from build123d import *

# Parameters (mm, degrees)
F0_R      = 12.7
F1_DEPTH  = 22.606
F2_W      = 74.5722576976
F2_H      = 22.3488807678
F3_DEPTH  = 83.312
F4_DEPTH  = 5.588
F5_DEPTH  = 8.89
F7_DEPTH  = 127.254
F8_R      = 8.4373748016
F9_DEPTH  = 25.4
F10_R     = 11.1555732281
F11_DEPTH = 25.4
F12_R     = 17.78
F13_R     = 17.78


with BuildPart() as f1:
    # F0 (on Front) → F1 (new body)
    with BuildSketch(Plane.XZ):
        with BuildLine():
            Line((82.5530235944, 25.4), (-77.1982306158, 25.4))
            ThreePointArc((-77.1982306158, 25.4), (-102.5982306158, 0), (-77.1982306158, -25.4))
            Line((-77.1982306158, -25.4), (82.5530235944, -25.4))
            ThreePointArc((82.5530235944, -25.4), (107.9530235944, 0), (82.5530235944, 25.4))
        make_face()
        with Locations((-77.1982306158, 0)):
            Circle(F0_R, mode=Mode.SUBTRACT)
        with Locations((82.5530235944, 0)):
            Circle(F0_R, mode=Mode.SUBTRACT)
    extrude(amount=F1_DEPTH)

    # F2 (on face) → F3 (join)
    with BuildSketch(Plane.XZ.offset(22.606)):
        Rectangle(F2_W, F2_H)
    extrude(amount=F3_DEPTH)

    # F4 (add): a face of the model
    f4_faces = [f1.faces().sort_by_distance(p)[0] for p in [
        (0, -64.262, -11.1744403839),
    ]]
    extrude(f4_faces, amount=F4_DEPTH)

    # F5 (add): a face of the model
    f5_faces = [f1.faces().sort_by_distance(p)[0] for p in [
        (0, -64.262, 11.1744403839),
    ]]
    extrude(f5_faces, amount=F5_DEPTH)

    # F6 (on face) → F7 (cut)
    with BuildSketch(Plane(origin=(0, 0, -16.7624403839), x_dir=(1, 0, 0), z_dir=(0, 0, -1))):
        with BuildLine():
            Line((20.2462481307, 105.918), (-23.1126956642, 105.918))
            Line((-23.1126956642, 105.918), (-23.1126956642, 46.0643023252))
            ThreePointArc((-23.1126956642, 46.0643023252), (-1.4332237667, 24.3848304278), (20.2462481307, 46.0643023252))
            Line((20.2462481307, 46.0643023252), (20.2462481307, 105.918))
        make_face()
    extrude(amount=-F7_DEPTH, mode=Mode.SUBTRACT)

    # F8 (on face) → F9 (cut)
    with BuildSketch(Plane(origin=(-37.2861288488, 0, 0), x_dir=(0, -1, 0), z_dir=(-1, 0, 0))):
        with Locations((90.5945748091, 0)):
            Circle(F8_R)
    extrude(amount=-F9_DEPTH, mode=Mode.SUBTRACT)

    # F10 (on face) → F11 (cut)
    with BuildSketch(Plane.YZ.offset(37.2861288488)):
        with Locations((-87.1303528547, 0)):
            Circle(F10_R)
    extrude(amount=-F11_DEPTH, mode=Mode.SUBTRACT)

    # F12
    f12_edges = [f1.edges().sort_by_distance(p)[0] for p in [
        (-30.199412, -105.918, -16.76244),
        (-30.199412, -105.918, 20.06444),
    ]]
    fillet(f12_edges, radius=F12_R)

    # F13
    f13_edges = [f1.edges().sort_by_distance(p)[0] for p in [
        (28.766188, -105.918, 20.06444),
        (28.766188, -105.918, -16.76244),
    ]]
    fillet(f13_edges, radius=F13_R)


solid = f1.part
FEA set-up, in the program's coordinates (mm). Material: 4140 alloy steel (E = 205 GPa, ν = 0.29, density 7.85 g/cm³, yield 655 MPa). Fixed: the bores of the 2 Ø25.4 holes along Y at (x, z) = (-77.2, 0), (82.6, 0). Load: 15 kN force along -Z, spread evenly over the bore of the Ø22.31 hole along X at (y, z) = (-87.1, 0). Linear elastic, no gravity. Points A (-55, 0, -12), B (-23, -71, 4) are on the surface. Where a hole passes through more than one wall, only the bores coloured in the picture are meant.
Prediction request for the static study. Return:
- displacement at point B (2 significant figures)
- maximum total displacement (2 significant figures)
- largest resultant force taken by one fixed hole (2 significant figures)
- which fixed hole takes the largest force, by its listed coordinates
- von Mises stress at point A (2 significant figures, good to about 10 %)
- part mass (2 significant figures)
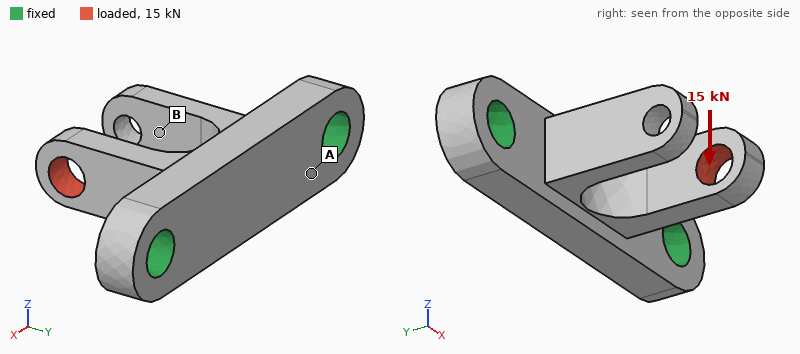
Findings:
0.083 mm
0.41 mm
11 kN
(82.6, 0)
74 MPa
2.3 kg
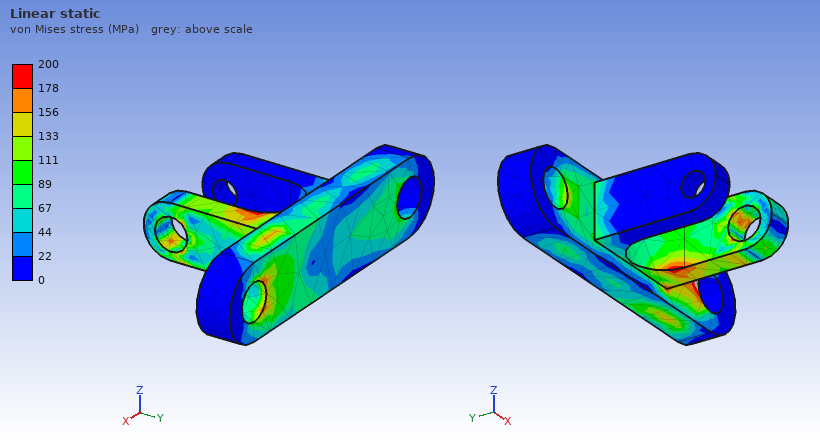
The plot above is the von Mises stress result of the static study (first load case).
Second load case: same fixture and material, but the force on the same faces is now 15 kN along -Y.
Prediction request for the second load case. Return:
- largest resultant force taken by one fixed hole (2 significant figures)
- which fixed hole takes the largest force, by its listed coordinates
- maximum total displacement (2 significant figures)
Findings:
11 kN
(82.6, 0)
34 µm
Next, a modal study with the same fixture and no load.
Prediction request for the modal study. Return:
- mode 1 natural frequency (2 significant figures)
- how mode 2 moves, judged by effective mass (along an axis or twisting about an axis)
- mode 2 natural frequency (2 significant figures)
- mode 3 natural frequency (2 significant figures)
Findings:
2200 Hz
along Z
2400 Hz
2700 Hz
